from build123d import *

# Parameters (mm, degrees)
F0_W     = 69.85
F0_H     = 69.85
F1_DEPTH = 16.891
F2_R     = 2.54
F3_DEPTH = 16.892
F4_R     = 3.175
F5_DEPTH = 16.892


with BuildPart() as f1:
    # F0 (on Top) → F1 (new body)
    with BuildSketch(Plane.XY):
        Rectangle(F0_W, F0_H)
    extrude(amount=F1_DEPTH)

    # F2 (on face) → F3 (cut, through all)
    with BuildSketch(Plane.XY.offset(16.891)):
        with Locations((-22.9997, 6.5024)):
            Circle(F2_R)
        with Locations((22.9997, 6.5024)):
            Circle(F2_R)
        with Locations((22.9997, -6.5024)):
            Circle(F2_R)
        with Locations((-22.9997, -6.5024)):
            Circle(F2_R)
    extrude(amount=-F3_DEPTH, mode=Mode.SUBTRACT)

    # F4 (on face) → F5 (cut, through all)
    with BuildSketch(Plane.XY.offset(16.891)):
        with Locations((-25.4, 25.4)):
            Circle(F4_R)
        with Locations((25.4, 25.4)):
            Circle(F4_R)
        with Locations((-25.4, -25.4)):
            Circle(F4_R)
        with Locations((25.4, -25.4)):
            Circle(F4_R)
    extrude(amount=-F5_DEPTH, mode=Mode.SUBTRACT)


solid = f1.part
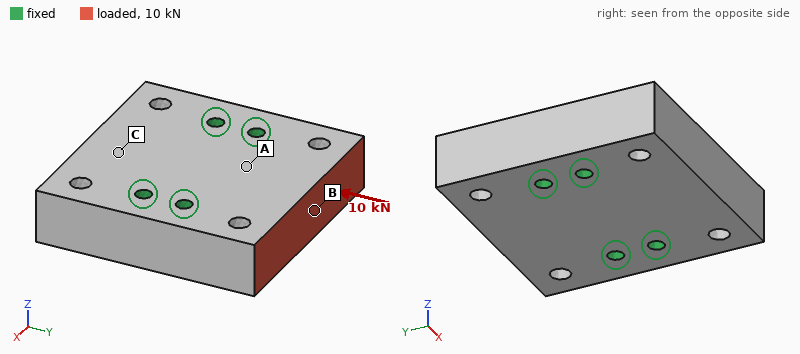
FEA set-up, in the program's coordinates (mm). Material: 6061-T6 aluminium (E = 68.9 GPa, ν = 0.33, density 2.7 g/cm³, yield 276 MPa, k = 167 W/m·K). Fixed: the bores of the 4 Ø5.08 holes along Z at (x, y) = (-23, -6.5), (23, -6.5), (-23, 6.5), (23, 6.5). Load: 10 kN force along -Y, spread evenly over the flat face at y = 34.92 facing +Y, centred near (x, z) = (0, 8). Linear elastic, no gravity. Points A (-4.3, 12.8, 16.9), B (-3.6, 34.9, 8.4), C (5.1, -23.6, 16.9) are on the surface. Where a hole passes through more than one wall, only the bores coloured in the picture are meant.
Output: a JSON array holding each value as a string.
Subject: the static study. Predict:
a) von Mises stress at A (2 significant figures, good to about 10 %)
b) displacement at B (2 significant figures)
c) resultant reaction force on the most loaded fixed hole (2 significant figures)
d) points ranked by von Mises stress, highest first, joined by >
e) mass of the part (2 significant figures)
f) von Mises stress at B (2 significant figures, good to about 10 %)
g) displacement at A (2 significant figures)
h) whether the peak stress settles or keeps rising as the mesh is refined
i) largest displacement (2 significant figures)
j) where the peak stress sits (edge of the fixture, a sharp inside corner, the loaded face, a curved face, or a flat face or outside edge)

["5.1 MPa", "4.7 µm", "3.5 kN", "B > A > C", "210 g", "7.7 MPa", "2.6 µm", "keeps rising", "5.4 µm", "edge of the fixture"]
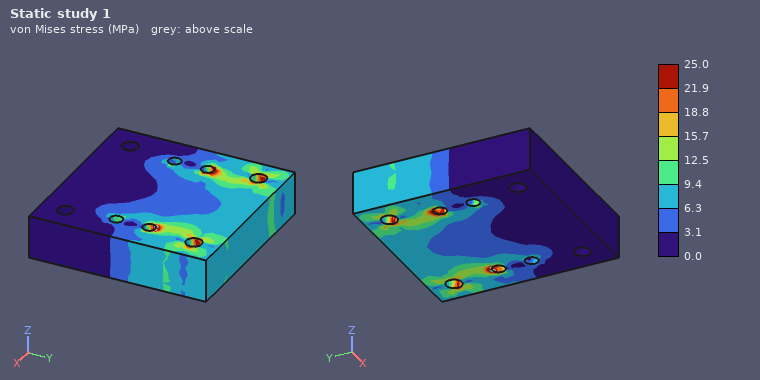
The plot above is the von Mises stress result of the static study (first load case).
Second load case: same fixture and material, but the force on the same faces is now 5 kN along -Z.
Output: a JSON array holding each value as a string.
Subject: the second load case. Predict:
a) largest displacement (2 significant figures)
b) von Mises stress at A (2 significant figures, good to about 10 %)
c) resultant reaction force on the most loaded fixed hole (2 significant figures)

["39 µm", "22 MPa", "3.5 kN"]
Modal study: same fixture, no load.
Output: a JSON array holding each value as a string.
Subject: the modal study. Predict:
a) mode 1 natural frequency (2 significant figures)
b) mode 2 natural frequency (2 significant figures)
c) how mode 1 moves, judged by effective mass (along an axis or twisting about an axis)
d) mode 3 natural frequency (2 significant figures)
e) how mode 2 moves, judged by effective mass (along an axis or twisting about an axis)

["11 kHz", "12 kHz", "twisting about X", "16 kHz", "along Z"]
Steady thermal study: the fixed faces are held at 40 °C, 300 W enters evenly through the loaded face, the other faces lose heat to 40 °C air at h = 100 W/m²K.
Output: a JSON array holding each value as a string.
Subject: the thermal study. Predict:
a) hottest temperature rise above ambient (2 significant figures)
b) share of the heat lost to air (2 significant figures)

["51 K", "5.9 %"]
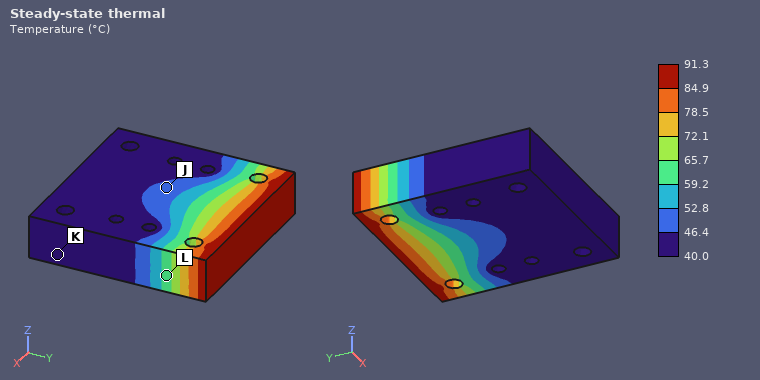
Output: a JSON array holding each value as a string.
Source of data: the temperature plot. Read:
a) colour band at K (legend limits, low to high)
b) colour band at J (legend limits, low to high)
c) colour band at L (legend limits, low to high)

["40.0 to 46.4 °C", "46.4 to 52.8 °C", "59.2 to 65.7 °C"]
